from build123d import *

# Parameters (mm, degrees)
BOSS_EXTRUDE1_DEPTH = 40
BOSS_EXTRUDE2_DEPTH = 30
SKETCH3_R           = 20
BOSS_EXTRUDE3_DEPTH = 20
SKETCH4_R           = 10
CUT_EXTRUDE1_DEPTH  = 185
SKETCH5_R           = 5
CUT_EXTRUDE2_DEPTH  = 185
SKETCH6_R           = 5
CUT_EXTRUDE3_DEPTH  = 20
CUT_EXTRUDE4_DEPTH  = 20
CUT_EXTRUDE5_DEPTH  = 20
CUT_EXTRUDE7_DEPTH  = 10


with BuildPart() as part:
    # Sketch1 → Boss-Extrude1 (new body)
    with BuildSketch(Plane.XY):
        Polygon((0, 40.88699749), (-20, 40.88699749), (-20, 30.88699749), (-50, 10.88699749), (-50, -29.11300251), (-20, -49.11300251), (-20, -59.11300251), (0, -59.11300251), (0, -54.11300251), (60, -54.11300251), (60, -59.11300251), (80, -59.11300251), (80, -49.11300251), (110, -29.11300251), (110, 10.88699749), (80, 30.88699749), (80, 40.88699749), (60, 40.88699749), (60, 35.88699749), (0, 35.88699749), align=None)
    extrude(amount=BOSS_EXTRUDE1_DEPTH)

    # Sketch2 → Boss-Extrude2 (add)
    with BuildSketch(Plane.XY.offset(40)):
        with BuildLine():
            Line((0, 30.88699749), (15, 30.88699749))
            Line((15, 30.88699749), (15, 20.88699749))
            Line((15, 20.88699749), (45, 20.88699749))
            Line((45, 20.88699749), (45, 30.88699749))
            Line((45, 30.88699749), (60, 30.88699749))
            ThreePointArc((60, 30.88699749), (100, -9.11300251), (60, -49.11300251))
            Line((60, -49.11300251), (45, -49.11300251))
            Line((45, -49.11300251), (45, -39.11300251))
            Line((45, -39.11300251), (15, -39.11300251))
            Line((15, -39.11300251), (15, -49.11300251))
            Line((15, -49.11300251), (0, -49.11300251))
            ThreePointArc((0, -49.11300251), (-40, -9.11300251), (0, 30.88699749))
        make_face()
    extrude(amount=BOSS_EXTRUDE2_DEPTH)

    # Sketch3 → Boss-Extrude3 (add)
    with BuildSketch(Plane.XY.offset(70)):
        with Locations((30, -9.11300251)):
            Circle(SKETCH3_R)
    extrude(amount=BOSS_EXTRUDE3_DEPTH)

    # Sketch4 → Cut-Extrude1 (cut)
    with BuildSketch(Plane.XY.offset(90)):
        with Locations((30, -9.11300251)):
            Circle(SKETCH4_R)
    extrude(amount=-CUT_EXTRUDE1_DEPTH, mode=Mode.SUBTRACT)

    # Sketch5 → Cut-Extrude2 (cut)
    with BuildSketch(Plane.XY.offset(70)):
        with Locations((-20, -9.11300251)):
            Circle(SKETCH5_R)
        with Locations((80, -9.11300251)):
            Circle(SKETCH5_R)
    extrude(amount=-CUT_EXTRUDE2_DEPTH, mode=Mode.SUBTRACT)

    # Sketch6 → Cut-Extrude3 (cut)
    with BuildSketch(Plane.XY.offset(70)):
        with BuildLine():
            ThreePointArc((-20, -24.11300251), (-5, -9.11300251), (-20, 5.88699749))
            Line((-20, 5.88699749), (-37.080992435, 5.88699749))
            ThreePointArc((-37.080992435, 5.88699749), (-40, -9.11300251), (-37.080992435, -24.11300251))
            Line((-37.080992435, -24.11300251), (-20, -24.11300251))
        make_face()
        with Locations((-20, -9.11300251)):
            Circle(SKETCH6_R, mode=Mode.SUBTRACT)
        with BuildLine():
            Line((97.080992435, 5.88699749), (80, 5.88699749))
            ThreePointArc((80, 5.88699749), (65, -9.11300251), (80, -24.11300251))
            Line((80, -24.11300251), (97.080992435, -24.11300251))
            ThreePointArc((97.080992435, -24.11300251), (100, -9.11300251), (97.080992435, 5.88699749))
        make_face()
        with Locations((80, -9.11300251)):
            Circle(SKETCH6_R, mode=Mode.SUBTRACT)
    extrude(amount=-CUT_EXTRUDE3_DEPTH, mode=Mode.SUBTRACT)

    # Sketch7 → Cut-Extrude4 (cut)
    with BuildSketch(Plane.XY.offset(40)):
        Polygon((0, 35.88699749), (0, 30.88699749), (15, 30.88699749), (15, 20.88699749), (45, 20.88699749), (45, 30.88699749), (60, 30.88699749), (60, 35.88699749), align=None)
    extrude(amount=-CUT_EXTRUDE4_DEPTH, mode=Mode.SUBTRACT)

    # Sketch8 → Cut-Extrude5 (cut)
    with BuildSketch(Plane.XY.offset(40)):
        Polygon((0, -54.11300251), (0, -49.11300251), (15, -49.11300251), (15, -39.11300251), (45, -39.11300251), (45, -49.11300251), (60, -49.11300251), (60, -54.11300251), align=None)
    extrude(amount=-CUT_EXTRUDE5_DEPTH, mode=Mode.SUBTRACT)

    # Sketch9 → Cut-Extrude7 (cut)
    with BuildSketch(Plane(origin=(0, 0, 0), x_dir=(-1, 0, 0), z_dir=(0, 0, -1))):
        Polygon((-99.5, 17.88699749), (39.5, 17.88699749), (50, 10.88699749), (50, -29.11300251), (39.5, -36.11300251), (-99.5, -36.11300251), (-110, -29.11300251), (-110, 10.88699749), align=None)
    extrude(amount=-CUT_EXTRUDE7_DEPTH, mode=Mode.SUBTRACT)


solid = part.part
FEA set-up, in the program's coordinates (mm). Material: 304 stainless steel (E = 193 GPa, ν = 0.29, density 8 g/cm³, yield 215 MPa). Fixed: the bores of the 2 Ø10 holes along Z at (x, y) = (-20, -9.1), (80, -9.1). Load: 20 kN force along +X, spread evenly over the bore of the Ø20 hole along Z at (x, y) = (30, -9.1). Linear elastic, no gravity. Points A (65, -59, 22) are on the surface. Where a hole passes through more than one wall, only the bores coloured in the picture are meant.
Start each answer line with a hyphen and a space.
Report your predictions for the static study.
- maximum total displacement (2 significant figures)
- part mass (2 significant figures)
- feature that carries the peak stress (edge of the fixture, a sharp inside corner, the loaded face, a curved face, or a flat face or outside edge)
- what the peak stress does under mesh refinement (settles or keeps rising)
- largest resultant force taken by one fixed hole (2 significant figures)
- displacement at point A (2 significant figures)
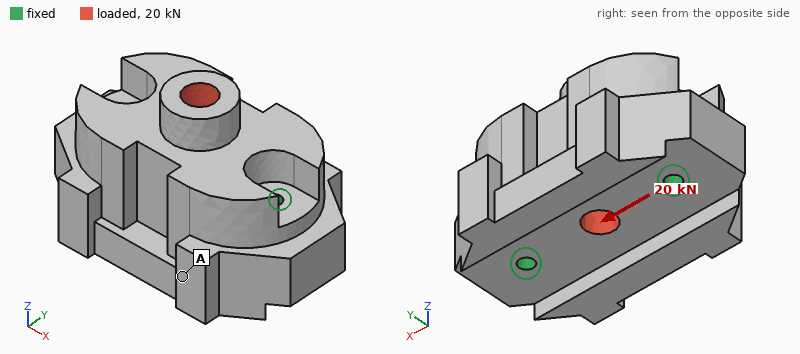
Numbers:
- 4.4 µm
- 5.2 kg
- edge of the fixture
- keeps rising
- 11 kN
- 0.85 µm
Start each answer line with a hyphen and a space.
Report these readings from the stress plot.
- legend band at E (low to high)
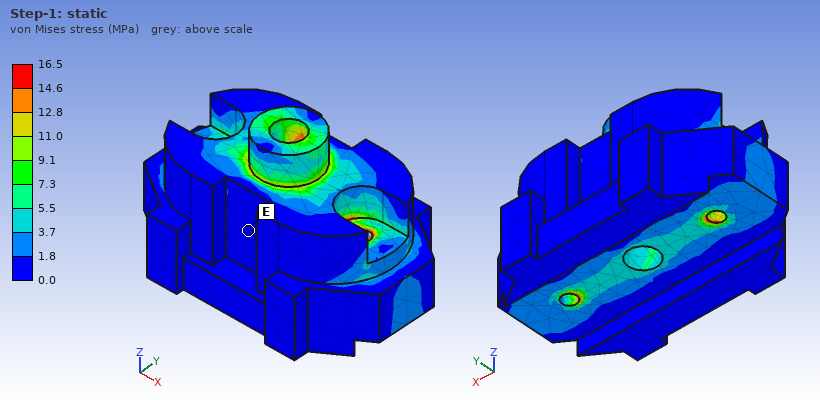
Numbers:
- 0.0 to 1.8 MPa
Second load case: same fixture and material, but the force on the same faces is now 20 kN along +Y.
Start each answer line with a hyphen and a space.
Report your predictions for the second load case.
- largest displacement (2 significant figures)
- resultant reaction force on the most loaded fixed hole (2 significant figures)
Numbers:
- 11 µm
- 10 kN
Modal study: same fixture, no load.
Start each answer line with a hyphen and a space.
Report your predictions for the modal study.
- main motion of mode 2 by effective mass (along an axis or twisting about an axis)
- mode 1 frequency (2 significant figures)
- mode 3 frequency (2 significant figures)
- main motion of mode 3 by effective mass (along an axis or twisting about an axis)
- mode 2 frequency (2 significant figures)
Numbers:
- along Z
- 5200 Hz
- 8800 Hz
- along Y
- 7800 Hz
